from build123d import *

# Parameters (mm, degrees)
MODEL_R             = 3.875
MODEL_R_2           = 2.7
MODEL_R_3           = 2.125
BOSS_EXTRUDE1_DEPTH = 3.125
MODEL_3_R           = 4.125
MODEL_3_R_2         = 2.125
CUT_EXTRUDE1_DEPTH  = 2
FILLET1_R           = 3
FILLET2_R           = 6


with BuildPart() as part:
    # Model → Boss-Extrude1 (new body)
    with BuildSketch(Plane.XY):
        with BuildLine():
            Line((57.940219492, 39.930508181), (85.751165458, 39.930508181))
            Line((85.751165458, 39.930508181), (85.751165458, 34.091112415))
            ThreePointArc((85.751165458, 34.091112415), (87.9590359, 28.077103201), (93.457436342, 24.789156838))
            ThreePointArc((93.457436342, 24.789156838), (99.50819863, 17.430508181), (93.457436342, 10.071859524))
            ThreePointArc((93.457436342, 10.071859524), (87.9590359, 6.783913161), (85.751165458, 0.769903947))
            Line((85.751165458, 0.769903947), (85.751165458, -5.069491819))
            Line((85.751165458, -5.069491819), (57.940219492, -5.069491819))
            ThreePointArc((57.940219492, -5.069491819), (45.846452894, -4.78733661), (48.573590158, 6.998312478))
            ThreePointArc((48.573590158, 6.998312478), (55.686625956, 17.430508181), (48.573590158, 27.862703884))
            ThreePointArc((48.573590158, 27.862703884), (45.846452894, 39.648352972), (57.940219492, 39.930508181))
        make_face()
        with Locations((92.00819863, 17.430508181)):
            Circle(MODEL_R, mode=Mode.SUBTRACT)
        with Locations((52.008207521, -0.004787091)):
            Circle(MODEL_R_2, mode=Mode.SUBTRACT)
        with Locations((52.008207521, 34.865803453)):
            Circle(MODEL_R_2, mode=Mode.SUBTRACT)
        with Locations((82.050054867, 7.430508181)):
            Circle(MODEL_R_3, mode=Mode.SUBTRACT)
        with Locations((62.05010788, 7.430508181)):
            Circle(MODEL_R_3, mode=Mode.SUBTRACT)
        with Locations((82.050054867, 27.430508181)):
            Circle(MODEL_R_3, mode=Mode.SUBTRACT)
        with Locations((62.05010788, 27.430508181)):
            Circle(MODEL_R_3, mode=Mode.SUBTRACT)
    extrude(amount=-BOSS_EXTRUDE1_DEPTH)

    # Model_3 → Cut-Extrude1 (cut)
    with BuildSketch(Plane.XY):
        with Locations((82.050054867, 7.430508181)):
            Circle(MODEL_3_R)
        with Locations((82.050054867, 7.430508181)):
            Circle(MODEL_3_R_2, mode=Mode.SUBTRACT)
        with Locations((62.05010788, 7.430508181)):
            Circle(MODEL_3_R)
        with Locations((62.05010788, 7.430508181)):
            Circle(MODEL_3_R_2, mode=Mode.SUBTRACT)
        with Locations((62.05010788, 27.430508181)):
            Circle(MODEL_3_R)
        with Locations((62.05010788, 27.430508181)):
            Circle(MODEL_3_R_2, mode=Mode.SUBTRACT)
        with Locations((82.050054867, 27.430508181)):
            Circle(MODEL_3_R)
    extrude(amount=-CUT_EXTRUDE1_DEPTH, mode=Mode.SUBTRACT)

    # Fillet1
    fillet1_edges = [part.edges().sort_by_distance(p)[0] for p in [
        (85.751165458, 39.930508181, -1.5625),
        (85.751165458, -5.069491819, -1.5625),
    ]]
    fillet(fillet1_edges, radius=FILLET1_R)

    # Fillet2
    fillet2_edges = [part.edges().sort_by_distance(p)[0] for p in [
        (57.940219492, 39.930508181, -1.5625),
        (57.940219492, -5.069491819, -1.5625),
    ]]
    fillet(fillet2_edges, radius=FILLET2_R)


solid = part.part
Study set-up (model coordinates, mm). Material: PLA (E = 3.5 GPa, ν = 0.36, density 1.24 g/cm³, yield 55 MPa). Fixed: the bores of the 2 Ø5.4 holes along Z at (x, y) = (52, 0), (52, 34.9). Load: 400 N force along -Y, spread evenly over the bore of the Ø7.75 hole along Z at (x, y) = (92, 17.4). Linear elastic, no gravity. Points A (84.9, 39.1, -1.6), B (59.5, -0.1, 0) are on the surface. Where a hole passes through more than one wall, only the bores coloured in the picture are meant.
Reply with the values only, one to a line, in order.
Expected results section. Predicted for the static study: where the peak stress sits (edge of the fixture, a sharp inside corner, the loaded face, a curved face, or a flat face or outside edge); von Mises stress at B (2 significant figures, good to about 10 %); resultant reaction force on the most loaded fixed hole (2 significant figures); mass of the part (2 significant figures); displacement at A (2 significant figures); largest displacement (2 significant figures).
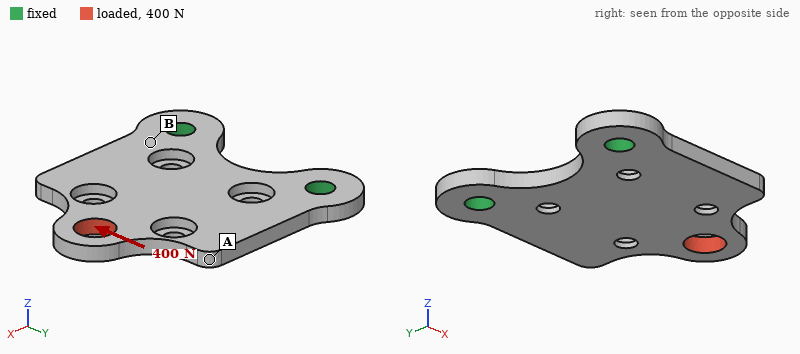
a curved face
13 MPa
460 N
6.4 g
0.23 mm
0.41 mm
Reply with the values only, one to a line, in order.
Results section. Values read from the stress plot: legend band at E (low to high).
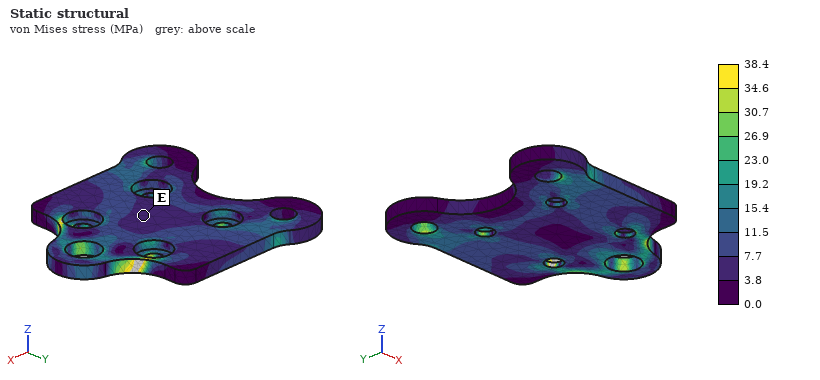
3.8 to 7.7 MPa
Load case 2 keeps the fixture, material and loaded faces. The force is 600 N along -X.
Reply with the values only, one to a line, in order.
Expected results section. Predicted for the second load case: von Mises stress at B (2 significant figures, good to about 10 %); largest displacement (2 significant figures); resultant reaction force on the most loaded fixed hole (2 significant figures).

10.0 MPa
0.32 mm
320 N
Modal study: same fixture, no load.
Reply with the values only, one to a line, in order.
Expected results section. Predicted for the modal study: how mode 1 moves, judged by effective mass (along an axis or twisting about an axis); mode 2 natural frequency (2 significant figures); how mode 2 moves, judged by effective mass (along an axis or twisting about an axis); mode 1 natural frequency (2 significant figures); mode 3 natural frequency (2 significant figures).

along Z
1500 Hz
twisting about X
530 Hz
2400 Hz
